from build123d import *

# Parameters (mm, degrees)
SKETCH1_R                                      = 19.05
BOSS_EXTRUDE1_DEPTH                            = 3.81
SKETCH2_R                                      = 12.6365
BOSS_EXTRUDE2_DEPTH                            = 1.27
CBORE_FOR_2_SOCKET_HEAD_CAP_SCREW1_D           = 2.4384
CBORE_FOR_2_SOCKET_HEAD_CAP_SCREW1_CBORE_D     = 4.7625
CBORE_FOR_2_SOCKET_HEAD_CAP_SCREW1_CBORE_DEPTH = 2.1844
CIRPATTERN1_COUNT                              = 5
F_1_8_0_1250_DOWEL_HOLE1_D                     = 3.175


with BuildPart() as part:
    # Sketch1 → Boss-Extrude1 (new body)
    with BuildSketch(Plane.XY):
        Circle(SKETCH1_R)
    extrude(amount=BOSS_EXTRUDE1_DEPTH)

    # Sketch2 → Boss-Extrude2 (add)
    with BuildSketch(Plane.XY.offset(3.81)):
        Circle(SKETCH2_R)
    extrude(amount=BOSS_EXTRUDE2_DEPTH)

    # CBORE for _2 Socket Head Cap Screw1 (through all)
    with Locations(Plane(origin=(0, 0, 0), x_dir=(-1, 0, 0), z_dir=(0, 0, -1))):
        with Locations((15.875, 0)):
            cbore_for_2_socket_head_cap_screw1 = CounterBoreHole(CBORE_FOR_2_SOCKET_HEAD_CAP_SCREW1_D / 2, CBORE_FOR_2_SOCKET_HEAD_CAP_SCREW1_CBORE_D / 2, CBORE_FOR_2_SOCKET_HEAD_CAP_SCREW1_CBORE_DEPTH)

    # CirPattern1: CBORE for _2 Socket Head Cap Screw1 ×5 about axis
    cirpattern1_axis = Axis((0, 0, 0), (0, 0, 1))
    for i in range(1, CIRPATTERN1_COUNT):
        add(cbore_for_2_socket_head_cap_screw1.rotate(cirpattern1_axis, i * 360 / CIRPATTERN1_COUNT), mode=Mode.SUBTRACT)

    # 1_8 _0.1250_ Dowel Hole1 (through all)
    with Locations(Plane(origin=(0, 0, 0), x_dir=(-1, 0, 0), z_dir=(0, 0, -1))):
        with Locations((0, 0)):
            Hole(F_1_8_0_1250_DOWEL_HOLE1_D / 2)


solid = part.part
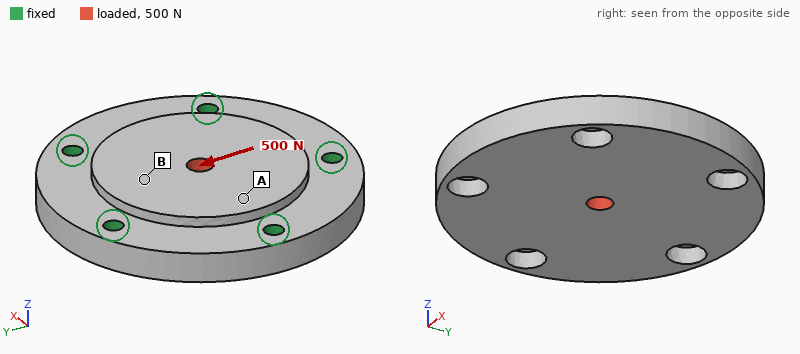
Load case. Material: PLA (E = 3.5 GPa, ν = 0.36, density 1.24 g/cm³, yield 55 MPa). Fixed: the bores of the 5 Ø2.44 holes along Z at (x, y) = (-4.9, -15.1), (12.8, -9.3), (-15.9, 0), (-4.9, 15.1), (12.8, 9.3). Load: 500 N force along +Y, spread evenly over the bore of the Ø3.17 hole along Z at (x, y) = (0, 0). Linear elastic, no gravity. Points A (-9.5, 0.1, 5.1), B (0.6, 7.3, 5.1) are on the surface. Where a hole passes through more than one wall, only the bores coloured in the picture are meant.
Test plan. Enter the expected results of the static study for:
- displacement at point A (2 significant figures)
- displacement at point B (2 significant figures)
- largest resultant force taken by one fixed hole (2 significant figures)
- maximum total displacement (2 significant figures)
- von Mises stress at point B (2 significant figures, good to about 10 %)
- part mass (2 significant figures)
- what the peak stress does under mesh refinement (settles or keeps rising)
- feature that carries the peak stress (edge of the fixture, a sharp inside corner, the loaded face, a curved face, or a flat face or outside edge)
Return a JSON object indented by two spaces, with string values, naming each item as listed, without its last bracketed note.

{
  "displacement at point A": "10 µm",
  "displacement at point B": "17 µm",
  "largest resultant force taken by one fixed hole": "130 N",
  "maximum total displacement": "28 µm",
  "von Mises stress at point B": "3.9 MPa",
  "part mass": "5.8 g",
  "what the peak stress does under mesh refinement": "keeps rising",
  "feature that carries the peak stress": "edge of the fixture"
}
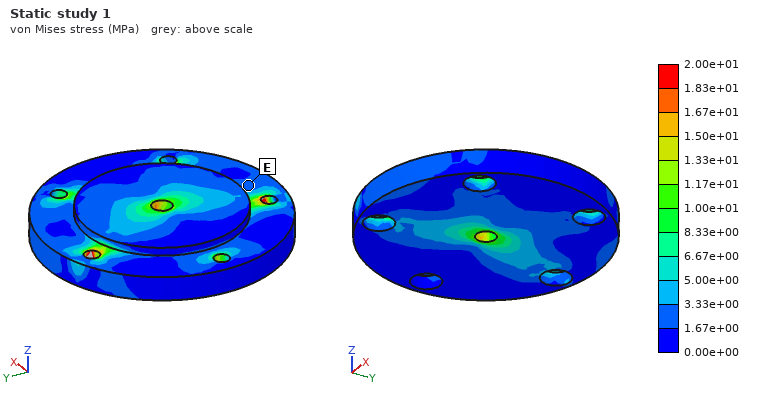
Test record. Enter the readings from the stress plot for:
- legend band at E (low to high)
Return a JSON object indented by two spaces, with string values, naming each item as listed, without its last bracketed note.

{
  "legend band at E": "1.67e+00 to 3.33e+00 MPa"
}
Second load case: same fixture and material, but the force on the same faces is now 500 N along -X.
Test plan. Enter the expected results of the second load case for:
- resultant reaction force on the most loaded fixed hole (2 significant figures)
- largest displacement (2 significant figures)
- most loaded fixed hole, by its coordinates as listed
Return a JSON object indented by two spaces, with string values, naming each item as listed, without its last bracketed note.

{
  "resultant reaction force on the most loaded fixed hole": "130 N",
  "largest displacement": "28 µm",
  "most loaded fixed hole, by its coordinates as listed": "(-15.9, 0)"
}
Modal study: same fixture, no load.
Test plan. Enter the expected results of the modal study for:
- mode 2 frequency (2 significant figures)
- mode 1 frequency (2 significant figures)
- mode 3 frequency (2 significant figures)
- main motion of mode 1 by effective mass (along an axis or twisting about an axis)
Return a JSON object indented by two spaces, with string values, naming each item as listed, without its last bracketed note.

{
  "mode 2 frequency": "10 kHz",
  "mode 1 frequency": "7600 Hz",
  "mode 3 frequency": "10 kHz",
  "main motion of mode 1 by effective mass": "along Z"
}
